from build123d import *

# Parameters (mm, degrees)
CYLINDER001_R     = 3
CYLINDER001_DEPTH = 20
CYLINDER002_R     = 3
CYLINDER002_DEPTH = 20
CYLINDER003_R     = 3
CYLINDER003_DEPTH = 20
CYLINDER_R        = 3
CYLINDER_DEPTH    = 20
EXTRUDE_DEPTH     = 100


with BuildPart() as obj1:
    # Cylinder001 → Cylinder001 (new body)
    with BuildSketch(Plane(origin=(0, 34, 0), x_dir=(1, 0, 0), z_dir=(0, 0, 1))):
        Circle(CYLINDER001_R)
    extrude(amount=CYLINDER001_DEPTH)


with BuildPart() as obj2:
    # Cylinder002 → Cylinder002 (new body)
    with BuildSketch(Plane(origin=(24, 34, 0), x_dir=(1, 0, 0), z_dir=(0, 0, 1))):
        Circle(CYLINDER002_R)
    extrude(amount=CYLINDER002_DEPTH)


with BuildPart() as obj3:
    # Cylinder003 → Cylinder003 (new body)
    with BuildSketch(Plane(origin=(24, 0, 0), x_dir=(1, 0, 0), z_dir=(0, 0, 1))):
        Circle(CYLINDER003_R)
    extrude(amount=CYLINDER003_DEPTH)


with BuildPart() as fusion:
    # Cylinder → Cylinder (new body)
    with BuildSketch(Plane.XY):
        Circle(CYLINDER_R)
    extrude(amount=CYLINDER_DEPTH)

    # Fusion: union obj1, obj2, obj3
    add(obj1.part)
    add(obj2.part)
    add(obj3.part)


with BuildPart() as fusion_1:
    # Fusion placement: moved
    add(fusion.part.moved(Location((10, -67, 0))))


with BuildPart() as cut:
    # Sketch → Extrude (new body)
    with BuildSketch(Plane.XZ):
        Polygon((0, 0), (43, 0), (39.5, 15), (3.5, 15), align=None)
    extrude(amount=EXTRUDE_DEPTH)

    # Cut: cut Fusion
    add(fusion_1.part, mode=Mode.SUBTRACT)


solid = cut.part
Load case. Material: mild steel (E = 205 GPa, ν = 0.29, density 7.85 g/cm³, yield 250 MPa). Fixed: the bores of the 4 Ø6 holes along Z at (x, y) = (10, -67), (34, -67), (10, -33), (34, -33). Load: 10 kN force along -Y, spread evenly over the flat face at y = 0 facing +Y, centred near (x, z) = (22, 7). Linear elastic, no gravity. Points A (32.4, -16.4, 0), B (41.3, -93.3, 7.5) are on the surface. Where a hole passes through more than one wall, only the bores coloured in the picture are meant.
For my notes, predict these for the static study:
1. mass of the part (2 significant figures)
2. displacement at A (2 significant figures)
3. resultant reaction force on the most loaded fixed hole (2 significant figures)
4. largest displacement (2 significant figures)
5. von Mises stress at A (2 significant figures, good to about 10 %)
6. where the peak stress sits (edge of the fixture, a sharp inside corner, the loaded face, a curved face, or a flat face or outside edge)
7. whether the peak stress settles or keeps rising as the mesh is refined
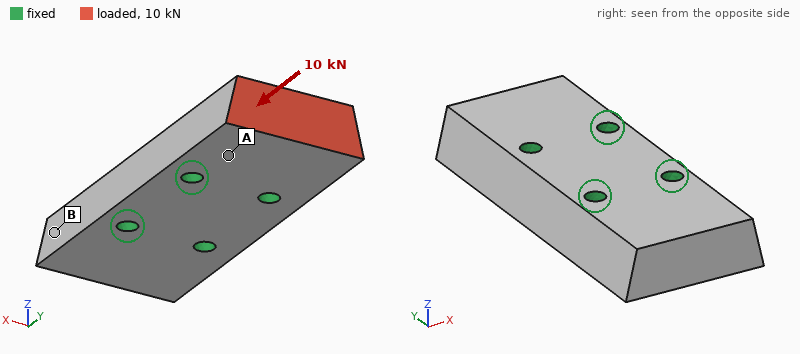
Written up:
450 g
1.5 µm
4.8 kN
2.9 µm
18 MPa
edge of the fixture
keeps rising
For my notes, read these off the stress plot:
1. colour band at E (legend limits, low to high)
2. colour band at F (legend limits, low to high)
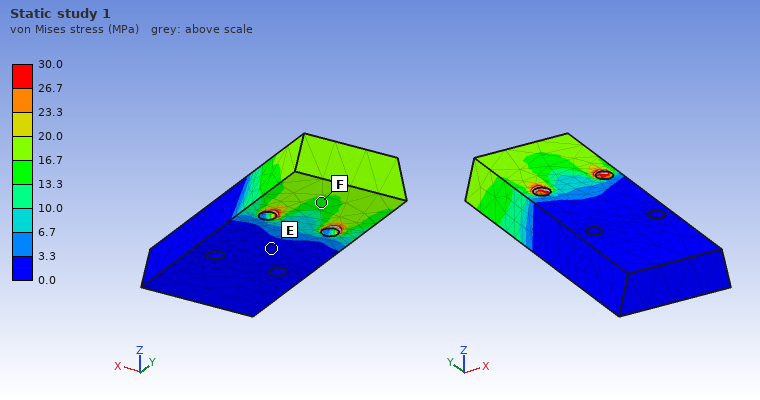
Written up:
0.0 to 3.3 MPa
13.3 to 16.7 MPa
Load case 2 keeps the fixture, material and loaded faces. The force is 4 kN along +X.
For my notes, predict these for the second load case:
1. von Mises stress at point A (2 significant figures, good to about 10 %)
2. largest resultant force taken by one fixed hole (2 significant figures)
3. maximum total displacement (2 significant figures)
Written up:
16 MPa
4.8 kN
7.9 µm
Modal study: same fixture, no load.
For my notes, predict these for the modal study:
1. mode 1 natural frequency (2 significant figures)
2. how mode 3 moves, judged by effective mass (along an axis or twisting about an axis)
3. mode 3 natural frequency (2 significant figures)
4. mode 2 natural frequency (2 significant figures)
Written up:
10000 Hz
twisting about Z
17 kHz
10 kHz
